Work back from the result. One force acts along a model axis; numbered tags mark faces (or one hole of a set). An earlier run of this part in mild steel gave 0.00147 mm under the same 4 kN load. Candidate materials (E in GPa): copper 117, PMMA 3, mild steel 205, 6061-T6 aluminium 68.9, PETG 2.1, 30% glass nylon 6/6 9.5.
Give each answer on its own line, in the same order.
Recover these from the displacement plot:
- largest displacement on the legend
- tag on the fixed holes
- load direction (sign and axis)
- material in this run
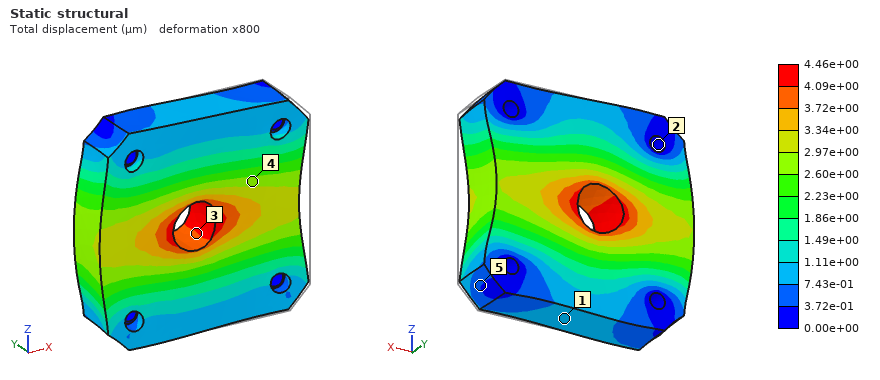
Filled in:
4.46e+00 µm
2
-X
6061-T6 aluminium
